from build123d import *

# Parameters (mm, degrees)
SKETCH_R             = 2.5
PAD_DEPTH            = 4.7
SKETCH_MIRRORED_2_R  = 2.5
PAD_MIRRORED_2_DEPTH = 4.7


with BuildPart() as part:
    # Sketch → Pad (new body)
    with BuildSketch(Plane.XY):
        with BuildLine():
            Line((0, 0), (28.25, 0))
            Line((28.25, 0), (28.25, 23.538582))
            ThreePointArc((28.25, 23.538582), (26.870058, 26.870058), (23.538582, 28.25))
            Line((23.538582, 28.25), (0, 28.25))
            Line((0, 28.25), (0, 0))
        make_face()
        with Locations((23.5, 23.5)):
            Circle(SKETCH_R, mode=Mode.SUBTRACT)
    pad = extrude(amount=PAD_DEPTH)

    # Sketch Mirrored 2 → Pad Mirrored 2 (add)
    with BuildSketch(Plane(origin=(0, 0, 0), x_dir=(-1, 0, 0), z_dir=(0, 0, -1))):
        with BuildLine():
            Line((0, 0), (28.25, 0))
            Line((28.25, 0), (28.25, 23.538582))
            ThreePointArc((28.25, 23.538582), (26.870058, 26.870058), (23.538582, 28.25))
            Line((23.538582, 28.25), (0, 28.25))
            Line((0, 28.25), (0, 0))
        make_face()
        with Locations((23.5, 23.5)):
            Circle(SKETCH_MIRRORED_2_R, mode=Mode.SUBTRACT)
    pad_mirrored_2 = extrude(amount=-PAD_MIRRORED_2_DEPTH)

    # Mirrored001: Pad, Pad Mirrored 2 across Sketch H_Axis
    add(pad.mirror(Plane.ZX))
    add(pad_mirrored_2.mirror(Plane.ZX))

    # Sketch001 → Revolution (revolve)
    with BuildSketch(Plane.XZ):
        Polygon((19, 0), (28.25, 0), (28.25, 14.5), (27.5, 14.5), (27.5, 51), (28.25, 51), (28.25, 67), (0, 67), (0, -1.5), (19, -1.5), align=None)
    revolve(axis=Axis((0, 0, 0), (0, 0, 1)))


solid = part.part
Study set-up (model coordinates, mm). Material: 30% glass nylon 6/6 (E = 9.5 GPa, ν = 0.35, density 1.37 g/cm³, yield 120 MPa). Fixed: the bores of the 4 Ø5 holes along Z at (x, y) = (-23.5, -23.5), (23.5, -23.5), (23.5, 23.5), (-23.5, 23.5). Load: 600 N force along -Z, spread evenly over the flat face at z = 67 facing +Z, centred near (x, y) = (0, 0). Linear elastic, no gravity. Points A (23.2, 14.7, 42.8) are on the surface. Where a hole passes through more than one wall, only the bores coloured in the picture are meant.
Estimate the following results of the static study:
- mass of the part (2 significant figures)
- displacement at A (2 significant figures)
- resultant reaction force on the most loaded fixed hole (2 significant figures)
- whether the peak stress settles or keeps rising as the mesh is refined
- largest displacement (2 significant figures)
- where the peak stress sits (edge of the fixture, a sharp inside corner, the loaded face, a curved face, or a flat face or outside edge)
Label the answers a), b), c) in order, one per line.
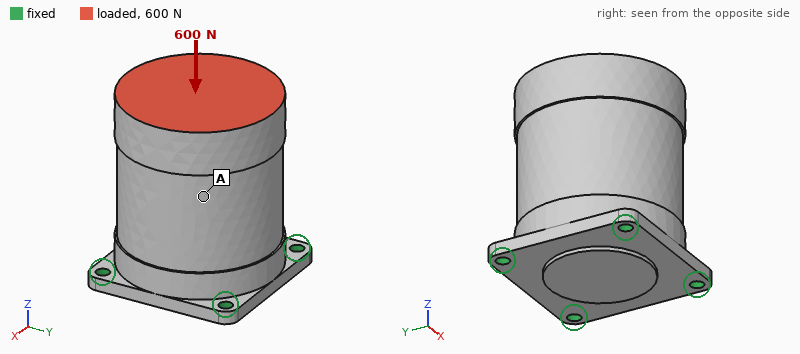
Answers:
a) 230 g
b) 8.7 µm
c) 160 N
d) keeps rising
e) 9.3 µm
f) edge of the fixture
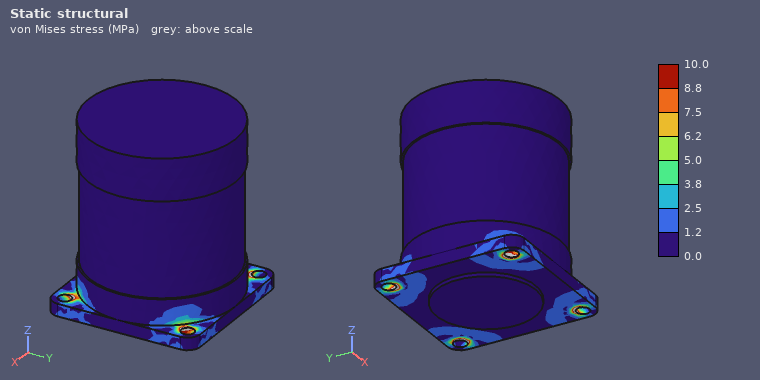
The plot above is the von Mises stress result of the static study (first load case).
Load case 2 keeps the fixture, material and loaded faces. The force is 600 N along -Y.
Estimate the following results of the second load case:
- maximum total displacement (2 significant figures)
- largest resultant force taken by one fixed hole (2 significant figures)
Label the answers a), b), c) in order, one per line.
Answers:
a) 94 µm
b) 500 N
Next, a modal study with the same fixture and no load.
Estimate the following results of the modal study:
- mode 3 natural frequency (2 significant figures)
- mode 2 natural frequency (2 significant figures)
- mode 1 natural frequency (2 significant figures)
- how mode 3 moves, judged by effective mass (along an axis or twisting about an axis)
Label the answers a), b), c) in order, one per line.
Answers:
a) 2900 Hz
b) 1500 Hz
c) 1500 Hz
d) along Z
